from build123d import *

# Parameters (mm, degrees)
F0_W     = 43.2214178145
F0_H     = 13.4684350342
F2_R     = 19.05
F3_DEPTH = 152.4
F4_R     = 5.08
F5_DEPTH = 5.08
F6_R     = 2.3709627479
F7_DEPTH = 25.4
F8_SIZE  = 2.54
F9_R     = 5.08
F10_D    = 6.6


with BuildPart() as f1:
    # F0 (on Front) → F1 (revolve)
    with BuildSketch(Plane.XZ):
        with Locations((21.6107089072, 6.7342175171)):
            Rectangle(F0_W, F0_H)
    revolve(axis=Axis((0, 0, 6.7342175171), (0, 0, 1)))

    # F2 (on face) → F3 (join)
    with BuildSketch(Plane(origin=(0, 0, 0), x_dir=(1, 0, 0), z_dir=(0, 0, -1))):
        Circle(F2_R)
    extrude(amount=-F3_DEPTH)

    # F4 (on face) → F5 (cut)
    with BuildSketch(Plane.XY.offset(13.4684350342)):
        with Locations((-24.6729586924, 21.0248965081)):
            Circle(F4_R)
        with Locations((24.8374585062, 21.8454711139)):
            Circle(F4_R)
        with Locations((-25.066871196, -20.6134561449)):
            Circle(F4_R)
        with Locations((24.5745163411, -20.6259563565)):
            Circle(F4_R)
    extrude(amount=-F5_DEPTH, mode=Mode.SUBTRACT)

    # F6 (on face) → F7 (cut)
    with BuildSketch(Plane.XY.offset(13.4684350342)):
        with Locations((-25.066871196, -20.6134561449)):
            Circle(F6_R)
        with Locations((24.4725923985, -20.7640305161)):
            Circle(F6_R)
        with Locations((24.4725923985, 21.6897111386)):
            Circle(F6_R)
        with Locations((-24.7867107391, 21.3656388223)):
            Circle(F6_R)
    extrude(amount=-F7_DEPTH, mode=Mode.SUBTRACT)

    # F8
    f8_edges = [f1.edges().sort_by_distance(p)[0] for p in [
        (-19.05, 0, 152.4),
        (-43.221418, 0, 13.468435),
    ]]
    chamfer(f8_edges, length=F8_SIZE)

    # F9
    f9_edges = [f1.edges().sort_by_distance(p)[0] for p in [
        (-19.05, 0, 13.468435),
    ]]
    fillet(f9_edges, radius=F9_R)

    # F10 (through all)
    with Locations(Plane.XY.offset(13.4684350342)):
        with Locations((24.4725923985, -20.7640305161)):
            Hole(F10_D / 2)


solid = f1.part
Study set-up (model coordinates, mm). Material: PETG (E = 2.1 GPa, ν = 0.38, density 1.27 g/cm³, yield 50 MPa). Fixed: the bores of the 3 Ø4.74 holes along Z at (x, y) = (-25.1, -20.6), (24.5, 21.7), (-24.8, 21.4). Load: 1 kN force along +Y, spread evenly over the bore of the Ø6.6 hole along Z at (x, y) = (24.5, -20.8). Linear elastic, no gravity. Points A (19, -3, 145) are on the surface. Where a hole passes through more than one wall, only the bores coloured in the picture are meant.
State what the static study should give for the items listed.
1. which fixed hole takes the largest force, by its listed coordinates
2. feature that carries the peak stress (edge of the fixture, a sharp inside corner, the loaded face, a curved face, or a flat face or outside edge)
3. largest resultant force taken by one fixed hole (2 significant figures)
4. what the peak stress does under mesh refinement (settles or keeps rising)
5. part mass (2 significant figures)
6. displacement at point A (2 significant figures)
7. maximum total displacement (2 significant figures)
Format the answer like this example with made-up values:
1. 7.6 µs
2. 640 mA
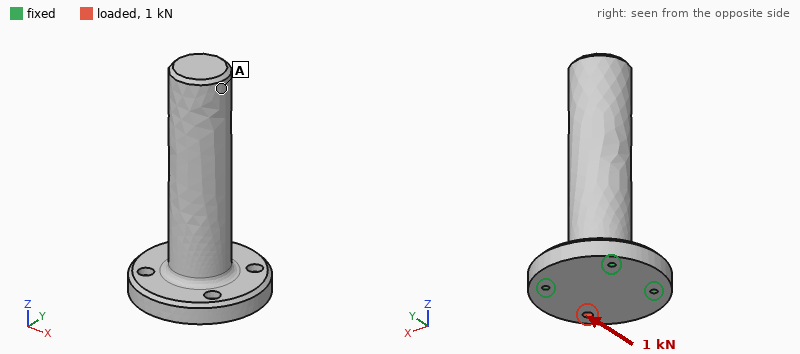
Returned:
1. (24.5, 21.7)
2. edge of the fixture
3. 790 N
4. keeps rising
5. 300 g
6. 0.035 mm
7. 0.12 mm
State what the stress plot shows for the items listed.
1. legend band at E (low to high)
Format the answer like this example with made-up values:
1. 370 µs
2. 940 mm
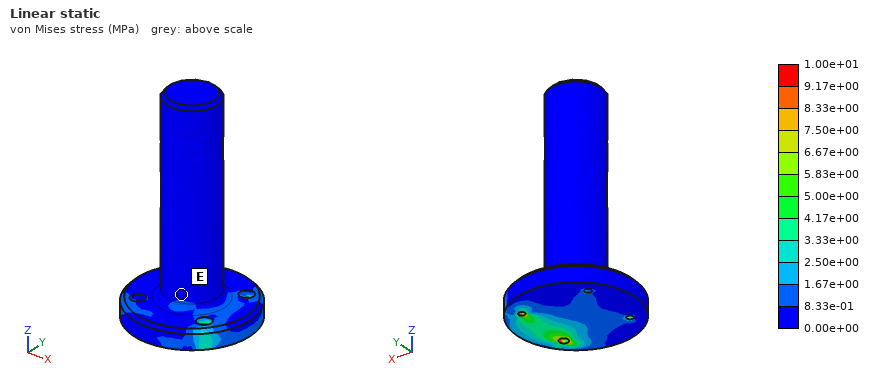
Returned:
1. 0.00e+00 to 8.33e-01 MPa
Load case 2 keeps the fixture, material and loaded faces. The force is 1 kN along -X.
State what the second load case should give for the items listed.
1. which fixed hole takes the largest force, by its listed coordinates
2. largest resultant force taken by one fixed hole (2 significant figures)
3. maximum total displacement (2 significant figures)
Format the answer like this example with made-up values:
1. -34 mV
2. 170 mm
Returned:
1. (-25.1, -20.6)
2. 700 N
3. 0.12 mm
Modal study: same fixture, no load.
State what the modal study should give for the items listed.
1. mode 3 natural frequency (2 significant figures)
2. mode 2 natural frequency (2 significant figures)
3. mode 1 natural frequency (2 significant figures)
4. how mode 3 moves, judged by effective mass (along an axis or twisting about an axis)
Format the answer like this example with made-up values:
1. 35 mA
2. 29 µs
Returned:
1. 1100 Hz
2. 280 Hz
3. 210 Hz
4. along Z
